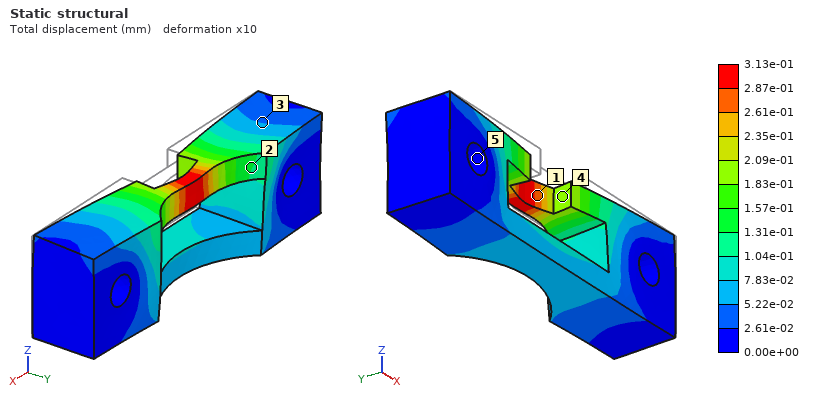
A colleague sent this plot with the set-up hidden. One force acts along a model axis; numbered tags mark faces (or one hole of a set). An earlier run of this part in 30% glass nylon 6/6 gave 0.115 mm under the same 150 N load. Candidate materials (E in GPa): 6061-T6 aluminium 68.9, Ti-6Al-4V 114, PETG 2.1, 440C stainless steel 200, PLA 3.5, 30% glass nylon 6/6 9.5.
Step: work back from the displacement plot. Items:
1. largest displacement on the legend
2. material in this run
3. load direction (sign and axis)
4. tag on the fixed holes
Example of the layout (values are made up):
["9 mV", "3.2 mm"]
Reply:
["3.13e-01 mm", "PLA", "+Y", "5"]
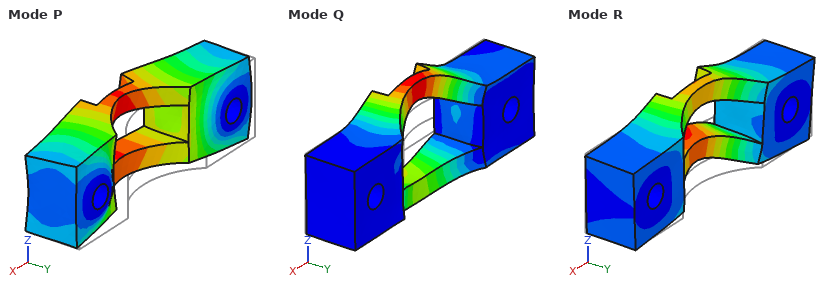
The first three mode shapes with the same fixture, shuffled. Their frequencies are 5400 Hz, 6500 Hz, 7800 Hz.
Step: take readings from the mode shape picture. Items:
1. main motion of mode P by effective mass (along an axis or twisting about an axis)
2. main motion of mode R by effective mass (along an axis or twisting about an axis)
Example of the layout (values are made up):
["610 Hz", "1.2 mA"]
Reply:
["along Y", "along Z"]
